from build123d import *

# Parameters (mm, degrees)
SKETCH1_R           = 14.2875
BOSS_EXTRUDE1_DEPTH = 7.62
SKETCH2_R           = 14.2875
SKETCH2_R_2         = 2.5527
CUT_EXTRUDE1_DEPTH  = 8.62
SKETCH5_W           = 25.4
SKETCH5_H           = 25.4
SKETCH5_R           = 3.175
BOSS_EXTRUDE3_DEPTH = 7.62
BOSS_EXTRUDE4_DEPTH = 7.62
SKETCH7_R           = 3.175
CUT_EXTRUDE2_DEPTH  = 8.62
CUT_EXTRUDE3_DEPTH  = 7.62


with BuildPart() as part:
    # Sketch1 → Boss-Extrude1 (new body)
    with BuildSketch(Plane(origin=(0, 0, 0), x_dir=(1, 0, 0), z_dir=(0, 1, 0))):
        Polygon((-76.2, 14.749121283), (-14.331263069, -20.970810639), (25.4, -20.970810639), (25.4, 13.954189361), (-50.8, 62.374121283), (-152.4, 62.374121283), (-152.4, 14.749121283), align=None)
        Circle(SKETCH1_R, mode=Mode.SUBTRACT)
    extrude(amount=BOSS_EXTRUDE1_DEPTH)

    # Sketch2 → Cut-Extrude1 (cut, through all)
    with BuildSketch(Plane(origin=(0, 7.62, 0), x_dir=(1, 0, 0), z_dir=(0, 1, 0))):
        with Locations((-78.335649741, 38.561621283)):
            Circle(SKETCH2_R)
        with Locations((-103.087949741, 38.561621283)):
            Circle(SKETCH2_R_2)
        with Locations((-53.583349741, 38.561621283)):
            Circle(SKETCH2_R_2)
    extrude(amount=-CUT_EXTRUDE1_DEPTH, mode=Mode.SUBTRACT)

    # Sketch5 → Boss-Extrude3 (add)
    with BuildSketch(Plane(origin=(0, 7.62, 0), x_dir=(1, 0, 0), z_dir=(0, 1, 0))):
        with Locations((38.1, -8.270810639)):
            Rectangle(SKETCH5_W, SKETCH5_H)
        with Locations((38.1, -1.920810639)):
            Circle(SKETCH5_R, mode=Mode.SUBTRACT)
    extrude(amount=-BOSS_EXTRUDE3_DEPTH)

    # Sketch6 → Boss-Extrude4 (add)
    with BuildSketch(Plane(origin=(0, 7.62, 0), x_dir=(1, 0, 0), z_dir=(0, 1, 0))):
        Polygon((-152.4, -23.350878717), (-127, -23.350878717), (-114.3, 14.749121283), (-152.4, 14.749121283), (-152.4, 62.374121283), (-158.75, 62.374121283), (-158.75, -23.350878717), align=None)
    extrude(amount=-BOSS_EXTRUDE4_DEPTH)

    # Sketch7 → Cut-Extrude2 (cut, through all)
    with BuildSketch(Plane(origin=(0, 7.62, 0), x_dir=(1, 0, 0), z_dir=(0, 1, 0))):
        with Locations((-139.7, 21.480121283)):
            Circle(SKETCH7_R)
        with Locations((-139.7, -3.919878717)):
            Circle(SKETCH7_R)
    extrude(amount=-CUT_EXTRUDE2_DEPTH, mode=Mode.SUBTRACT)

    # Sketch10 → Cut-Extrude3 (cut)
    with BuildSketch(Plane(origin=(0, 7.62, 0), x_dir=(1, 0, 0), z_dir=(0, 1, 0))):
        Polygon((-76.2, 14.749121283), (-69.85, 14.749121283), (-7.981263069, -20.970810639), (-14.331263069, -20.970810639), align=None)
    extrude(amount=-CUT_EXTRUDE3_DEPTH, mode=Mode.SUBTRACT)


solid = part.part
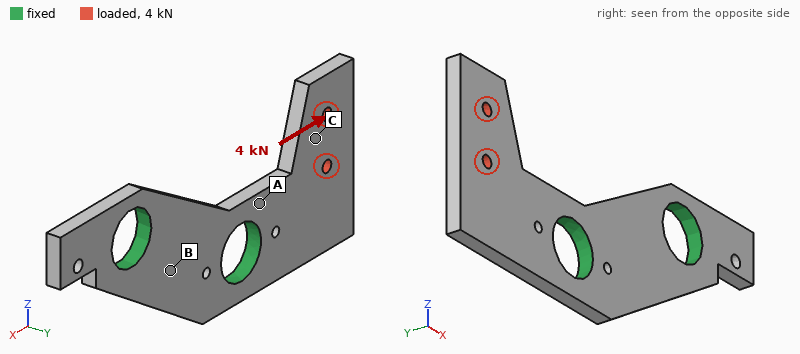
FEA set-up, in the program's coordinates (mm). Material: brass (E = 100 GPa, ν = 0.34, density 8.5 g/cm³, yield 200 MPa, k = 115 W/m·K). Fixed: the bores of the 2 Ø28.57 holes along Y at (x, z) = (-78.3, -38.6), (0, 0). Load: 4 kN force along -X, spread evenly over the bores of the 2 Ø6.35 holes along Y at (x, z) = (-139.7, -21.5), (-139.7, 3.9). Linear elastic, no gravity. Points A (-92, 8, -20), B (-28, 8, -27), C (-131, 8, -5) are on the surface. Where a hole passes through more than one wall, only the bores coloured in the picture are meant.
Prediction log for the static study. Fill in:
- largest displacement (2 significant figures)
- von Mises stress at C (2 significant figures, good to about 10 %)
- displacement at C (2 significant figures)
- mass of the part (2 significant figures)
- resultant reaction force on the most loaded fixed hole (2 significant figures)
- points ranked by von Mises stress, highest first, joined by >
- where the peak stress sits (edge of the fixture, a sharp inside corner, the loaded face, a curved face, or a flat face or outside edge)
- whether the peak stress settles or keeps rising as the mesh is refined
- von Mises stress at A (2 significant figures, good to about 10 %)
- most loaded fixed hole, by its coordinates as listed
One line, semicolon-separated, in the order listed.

84 µm; 16 MPa; 45 µm; 640 g; 3.9 kN; A > C > B; a sharp inside corner; keeps rising; 37 MPa; (-78.3, -38.6)
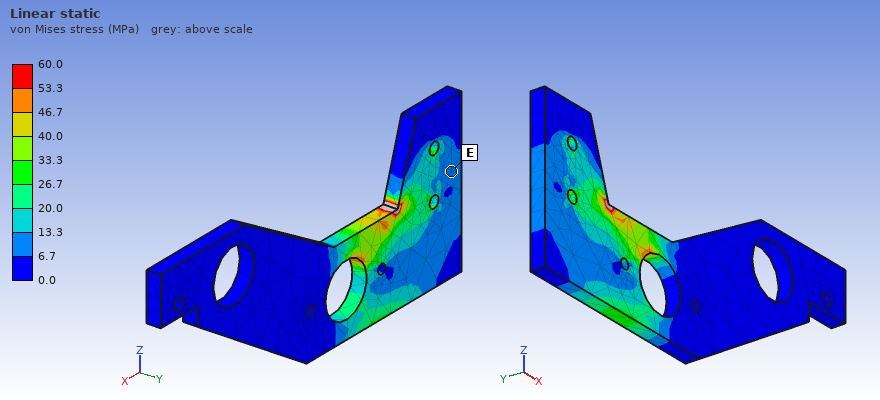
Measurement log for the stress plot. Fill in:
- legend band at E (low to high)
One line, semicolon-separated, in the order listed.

6.7 to 13.3 MPa
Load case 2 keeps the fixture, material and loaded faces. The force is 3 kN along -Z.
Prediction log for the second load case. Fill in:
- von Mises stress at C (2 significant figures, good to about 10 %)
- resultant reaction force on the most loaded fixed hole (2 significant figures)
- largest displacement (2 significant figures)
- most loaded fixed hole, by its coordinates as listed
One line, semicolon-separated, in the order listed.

6.0 MPa; 3.2 kN; 82 µm; (-78.3, -38.6)
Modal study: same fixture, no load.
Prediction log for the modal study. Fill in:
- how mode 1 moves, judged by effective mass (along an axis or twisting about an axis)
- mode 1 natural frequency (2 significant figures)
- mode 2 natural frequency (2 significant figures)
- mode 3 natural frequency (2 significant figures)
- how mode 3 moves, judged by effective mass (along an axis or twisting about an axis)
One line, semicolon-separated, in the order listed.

along Y; 600 Hz; 1200 Hz; 2400 Hz; along Z
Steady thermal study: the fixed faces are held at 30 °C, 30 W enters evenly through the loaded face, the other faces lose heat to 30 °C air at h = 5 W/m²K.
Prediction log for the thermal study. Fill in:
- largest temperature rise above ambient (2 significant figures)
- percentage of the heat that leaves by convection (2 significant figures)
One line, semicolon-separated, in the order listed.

48 K; 5.4 %
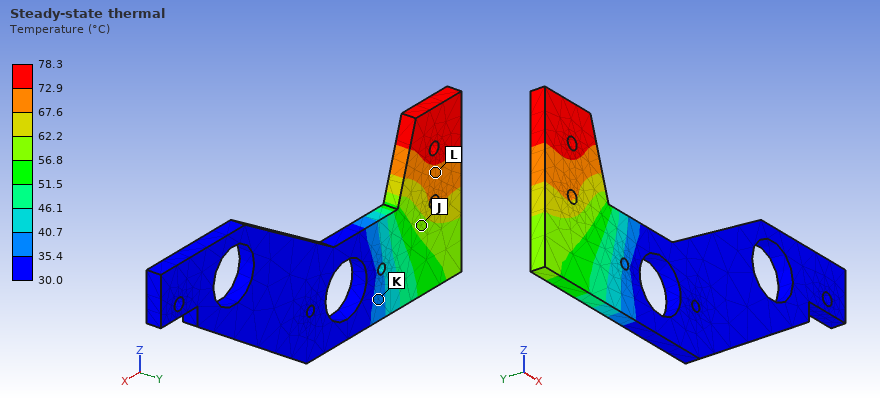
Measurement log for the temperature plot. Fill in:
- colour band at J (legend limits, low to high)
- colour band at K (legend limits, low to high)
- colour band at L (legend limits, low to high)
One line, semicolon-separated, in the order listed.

56.8 to 62.2 °C; 35.4 to 40.7 °C; 67.6 to 72.9 °C
